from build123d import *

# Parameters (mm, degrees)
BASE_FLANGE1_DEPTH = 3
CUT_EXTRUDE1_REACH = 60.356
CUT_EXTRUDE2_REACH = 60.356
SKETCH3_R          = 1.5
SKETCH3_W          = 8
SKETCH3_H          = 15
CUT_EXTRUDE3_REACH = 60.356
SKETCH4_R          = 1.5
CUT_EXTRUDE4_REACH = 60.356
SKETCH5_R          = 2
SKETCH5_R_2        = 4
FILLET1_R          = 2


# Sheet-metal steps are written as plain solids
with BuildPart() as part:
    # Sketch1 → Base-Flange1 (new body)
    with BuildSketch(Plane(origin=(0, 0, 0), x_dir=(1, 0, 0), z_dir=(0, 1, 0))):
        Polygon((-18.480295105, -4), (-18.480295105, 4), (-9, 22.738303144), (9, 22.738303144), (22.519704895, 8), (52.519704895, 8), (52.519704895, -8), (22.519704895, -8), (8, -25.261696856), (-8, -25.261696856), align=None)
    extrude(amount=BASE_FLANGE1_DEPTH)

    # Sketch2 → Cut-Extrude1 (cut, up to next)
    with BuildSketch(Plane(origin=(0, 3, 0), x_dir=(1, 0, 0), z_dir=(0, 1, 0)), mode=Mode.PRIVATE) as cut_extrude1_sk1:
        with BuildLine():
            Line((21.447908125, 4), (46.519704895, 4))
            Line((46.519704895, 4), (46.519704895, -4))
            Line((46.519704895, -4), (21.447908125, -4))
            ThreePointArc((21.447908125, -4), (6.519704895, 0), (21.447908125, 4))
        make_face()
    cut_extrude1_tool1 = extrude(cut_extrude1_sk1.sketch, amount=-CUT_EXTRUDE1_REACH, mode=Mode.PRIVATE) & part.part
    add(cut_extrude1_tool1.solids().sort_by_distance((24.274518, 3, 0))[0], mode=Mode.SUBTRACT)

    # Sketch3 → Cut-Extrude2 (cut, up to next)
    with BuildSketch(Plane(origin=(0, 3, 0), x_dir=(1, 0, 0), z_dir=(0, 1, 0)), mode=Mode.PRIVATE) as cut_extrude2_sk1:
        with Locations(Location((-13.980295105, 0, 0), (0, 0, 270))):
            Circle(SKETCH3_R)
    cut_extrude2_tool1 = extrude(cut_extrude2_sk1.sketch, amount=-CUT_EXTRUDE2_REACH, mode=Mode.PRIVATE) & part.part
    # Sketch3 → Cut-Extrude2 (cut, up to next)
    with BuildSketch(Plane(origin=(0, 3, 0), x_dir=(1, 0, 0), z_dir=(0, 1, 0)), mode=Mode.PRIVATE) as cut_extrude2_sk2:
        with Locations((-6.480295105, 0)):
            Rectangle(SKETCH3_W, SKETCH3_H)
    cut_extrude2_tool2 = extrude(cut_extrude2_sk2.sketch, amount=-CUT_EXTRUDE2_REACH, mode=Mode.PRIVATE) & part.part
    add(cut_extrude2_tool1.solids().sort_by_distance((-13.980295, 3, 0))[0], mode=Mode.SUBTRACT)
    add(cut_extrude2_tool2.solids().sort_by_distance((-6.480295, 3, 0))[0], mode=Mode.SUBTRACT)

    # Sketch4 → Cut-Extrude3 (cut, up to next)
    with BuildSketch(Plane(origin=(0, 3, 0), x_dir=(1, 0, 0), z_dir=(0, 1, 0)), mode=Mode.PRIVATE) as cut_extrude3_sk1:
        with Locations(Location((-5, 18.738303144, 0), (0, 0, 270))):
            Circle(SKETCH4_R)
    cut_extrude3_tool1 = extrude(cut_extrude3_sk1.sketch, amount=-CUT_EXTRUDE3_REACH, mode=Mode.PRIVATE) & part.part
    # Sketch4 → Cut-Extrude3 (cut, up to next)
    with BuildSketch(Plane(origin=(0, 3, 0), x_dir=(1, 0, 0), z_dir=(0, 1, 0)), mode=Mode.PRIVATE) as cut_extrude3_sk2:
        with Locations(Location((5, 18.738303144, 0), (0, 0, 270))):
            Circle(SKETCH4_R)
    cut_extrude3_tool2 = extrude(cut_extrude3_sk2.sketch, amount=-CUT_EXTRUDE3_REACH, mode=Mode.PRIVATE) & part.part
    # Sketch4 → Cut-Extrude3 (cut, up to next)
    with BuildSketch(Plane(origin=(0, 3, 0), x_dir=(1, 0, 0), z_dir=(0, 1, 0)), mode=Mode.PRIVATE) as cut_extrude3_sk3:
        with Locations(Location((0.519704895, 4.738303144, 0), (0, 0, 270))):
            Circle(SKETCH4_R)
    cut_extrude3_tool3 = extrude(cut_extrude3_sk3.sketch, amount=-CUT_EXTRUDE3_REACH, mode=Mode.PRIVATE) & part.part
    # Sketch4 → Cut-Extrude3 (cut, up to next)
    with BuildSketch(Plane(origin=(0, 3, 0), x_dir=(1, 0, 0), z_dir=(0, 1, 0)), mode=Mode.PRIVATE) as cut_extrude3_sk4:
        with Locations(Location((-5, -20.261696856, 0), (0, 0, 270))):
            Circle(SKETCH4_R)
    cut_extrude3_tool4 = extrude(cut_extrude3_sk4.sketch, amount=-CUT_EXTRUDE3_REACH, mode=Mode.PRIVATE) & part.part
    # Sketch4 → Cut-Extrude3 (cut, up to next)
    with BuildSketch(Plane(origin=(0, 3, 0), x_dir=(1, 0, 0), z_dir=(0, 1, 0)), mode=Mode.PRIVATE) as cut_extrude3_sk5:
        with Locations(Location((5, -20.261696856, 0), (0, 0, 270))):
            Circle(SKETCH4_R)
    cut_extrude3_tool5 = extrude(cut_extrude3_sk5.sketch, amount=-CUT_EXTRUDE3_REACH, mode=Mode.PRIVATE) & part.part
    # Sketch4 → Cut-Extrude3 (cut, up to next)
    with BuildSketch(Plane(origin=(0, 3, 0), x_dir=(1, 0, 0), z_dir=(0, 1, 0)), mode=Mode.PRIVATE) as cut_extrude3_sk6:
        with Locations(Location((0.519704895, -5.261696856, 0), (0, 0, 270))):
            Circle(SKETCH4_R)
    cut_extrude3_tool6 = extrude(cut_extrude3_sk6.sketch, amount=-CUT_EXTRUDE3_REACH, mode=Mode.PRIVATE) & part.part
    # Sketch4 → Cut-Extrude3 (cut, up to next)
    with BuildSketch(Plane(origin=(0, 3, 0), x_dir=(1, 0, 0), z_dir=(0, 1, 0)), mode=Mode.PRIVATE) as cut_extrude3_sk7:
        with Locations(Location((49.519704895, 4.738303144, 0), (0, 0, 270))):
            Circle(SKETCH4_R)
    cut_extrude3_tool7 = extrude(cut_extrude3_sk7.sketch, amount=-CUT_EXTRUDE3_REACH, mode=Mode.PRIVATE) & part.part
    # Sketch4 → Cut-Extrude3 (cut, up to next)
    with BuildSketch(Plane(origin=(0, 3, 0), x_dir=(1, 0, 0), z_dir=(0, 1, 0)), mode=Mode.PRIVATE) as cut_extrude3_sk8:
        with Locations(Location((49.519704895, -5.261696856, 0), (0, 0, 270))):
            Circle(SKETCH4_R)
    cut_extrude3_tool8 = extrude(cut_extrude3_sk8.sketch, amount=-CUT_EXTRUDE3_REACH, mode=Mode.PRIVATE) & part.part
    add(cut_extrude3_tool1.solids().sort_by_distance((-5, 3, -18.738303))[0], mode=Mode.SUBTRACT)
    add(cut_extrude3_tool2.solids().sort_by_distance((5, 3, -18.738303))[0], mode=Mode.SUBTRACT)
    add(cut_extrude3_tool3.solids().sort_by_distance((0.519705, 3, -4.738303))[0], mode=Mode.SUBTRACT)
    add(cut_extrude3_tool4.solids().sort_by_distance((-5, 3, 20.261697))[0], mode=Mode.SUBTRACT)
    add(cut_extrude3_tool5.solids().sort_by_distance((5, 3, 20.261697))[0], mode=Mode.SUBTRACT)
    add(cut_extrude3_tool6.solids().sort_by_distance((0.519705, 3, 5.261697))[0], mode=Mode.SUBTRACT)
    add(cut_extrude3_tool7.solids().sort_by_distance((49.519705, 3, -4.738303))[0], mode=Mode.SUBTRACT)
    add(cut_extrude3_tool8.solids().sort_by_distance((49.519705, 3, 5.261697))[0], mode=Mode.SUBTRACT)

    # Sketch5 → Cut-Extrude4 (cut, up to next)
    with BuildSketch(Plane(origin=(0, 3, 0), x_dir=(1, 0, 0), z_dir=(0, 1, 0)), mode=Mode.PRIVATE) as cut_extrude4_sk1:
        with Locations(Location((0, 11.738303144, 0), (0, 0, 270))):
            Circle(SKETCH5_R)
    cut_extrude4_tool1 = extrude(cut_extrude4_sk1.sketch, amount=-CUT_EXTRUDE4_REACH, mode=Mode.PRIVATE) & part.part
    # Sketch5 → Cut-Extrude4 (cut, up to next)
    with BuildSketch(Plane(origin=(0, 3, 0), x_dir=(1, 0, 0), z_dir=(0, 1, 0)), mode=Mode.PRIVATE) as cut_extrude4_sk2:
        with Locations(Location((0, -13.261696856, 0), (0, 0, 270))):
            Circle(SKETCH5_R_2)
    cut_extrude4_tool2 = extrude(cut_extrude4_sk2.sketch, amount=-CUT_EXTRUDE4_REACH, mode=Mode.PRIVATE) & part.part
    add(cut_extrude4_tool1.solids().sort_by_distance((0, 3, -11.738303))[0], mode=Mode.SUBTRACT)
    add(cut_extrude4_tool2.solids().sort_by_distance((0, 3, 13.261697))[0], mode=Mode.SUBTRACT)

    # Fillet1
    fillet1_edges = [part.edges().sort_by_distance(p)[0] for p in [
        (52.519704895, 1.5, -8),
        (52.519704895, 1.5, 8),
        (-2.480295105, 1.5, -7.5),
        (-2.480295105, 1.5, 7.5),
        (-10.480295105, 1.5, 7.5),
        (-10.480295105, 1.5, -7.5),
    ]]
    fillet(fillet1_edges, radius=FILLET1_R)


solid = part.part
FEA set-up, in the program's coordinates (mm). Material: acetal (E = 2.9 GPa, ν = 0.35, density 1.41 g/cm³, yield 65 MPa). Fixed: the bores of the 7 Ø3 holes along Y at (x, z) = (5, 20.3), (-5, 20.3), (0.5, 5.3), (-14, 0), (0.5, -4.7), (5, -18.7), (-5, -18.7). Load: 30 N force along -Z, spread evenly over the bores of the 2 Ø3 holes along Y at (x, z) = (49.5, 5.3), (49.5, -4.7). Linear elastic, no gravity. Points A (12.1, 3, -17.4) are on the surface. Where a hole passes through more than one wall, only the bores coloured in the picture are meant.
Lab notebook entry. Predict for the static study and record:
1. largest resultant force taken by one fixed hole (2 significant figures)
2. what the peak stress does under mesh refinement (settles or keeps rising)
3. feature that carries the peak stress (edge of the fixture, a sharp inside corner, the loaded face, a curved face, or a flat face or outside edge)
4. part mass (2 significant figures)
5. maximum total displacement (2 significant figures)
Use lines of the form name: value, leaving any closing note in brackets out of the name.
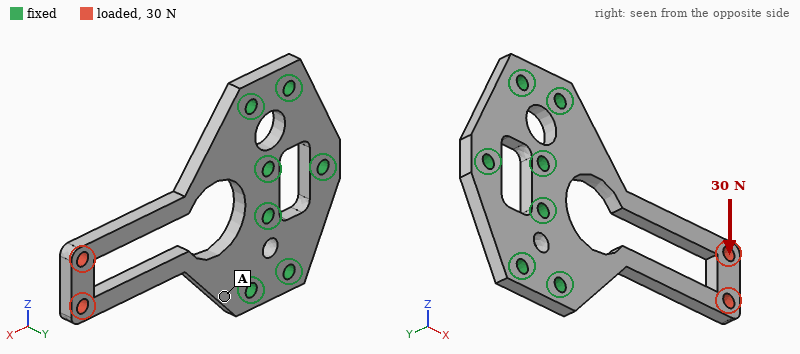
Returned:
largest resultant force taken by one fixed hole: 33 N
what the peak stress does under mesh refinement: keeps rising
feature that carries the peak stress: a sharp inside corner
part mass: 5.8 g
maximum total displacement: 0.92 mm
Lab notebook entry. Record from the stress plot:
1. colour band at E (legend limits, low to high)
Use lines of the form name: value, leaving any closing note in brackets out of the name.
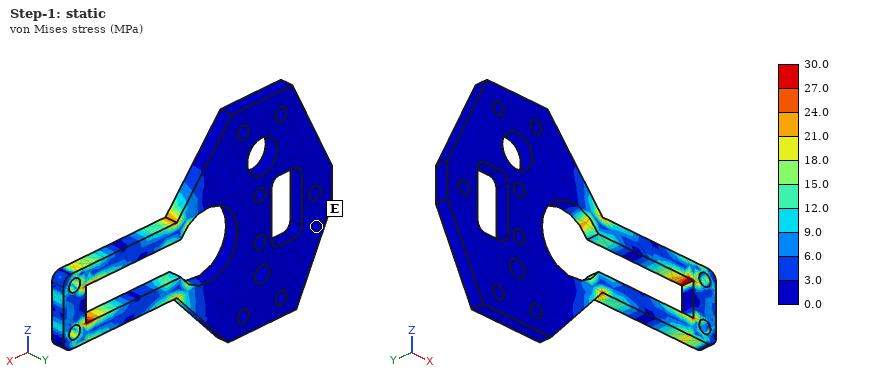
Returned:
colour band at E: 0.0 to 3.0 MPa
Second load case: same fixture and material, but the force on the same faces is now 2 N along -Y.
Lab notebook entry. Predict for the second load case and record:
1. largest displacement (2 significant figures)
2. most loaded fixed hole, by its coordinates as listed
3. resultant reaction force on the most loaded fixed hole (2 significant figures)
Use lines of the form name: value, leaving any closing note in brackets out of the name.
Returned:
largest displacement: 0.89 mm
most loaded fixed hole, by its coordinates as listed: (5, -18.7)
resultant reaction force on the most loaded fixed hole: 1.9 N
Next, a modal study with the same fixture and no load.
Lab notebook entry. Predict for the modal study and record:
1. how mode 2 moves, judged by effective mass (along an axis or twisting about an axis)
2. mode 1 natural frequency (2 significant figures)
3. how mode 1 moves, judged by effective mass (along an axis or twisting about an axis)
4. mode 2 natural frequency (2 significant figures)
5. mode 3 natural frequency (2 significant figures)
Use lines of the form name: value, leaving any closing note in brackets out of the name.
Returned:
how mode 2 moves, judged by effective mass: along Z
mode 1 natural frequency: 330 Hz
how mode 1 moves, judged by effective mass: along Y
mode 2 natural frequency: 1100 Hz
mode 3 natural frequency: 1300 Hz
